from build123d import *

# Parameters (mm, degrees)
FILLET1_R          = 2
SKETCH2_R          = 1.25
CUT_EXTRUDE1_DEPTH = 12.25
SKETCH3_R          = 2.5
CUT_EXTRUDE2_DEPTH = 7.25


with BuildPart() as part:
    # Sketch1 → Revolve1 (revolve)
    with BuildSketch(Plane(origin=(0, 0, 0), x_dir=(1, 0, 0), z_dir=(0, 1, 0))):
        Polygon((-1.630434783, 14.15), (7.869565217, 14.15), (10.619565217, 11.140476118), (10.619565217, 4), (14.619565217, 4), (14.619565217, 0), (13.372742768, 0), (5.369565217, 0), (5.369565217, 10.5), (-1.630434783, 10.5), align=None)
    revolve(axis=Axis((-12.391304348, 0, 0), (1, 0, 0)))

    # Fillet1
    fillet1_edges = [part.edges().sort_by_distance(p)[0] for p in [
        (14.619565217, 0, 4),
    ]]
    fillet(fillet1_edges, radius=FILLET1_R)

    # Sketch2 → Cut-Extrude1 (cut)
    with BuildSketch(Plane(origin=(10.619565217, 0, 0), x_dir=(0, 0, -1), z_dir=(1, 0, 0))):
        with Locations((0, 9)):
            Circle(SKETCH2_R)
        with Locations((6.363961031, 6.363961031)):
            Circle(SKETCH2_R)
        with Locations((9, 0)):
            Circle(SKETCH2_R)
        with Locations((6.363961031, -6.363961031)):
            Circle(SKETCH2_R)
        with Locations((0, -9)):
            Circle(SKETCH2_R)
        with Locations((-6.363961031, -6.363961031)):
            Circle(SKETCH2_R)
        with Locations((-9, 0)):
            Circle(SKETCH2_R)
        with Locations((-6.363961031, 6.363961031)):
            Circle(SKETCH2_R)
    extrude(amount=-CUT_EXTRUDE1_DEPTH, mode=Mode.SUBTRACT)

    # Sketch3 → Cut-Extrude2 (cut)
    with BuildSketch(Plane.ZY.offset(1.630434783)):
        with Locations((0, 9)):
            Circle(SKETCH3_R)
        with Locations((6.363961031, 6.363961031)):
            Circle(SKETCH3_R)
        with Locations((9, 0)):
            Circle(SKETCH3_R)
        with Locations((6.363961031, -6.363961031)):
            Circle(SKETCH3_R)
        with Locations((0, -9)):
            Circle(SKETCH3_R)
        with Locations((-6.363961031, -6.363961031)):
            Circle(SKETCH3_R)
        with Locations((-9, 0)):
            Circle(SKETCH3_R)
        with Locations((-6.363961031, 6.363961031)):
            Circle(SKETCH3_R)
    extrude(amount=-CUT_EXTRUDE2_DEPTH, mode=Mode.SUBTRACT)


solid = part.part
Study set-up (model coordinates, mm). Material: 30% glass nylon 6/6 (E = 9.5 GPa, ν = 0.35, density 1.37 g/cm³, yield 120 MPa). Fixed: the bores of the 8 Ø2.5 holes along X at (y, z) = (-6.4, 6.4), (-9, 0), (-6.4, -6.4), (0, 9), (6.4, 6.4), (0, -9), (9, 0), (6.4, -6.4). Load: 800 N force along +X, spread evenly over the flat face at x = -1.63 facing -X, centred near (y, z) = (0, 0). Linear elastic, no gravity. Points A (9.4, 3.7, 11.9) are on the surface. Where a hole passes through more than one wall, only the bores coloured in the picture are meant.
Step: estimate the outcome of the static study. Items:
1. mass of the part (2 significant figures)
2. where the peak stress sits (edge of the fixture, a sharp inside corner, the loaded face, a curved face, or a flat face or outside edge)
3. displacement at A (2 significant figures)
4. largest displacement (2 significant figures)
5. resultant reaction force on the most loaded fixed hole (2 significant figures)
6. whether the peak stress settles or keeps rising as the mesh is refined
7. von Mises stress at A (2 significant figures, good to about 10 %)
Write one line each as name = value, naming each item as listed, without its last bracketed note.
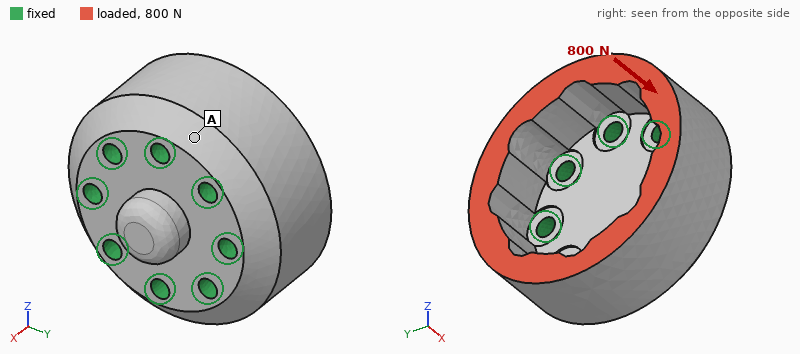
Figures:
mass of the part = 6.5 g
where the peak stress sits = edge of the fixture
displacement at A = 2.9 µm
largest displacement = 6.9 µm
resultant reaction force on the most loaded fixed hole = 100 N
whether the peak stress settles or keeps rising as the mesh is refined = keeps rising
von Mises stress at A = 1.7 MPa
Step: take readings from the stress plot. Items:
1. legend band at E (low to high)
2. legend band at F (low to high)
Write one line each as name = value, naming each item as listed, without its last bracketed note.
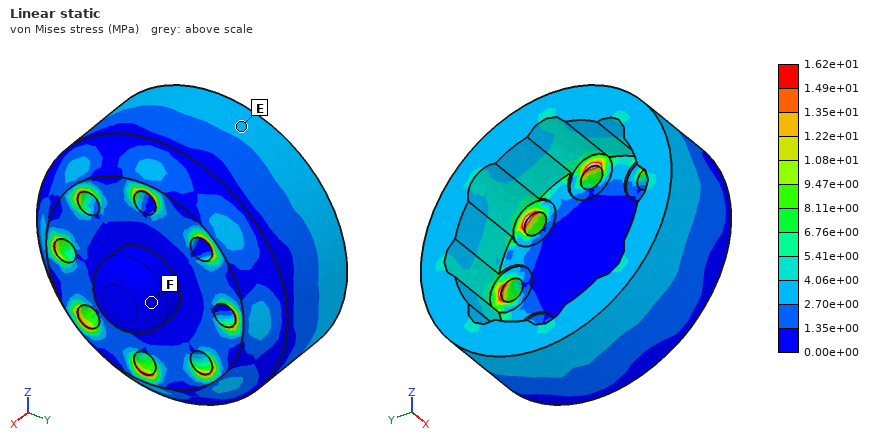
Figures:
legend band at E = 2.70e+00 to 4.06e+00 MPa
legend band at F = 0.00e+00 to 1.35e+00 MPa
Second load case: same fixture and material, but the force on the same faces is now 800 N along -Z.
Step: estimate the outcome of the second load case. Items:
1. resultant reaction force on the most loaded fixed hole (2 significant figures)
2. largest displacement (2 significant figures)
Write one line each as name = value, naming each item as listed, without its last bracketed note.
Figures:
resultant reaction force on the most loaded fixed hole = 190 N
largest displacement = 45 µm
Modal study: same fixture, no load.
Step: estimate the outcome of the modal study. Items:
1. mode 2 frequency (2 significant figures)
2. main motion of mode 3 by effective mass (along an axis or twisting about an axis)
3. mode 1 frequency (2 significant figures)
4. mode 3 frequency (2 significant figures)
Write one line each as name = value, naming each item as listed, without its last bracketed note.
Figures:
mode 2 frequency = 20 kHz
main motion of mode 3 by effective mass = along Y
mode 1 frequency = 20 kHz
mode 3 frequency = 22 kHz
